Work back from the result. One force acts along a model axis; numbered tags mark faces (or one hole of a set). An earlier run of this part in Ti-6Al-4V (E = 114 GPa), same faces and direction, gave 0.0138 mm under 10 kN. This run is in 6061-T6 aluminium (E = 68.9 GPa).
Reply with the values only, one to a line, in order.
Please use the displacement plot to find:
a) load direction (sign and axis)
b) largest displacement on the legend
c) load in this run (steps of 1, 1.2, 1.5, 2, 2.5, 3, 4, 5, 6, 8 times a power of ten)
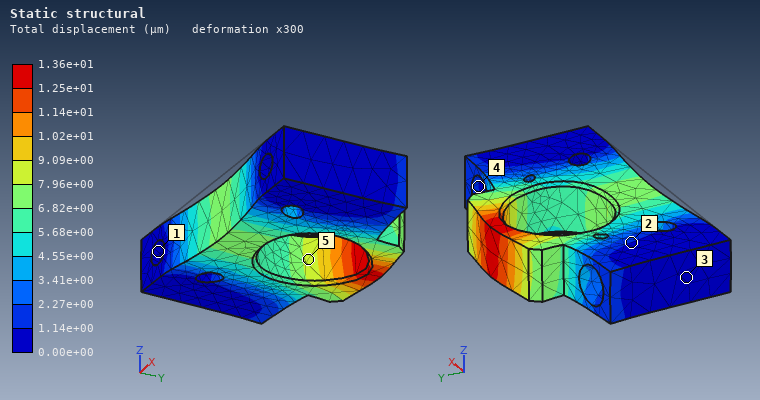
+Y
1.36e+01 µm
6 kN
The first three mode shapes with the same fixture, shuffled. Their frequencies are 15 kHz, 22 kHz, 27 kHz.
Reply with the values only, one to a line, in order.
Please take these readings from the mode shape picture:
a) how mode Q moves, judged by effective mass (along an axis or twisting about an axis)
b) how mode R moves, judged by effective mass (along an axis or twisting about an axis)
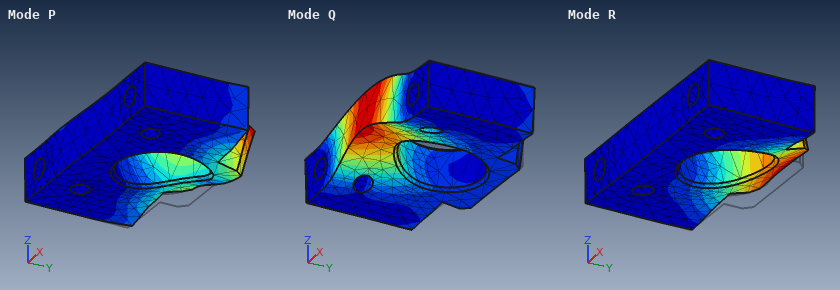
along Z
along Z
